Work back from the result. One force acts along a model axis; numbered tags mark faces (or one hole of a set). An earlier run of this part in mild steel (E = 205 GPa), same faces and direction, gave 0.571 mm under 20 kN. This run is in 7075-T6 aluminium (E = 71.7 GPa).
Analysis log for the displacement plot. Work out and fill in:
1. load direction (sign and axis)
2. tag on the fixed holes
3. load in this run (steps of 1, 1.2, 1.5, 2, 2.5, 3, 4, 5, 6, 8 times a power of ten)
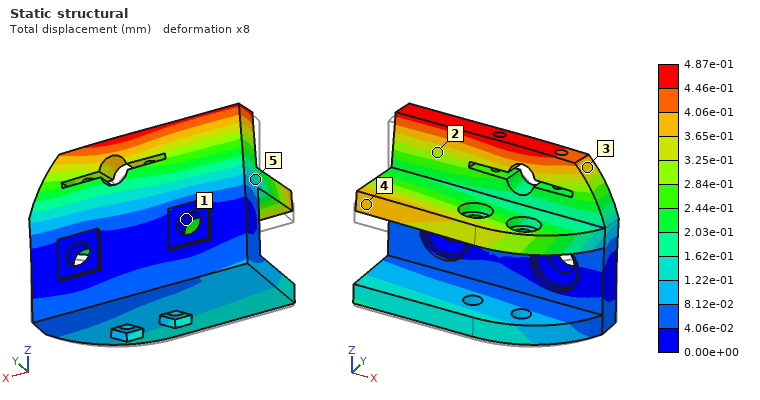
+Y
1
6 kN
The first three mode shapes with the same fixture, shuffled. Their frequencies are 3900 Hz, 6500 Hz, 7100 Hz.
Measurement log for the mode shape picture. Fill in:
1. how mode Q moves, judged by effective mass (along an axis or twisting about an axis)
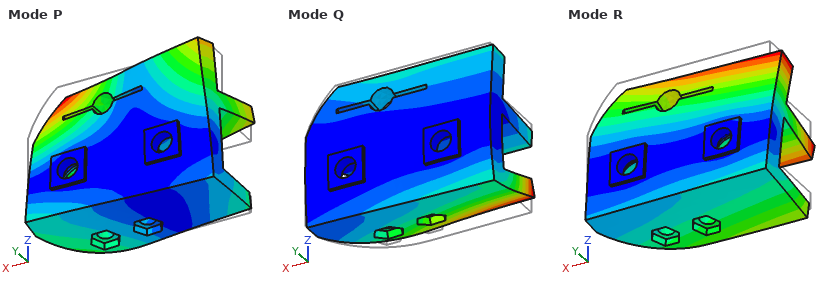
along Y
